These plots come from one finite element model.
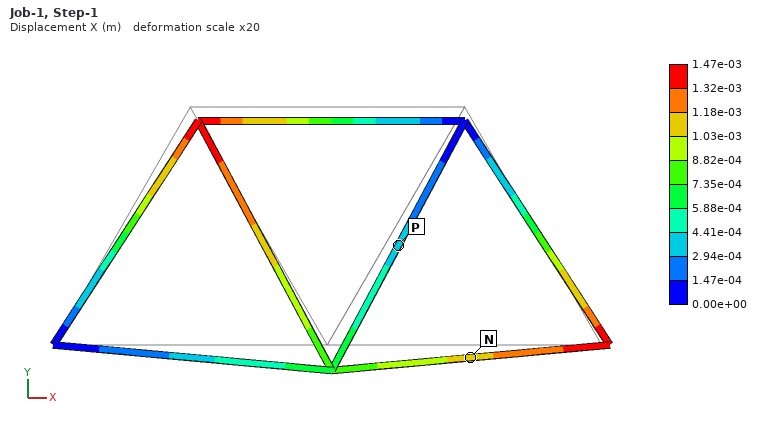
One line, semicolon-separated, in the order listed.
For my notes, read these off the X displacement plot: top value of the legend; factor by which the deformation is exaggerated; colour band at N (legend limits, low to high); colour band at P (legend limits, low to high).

1.47e-03 m; 20; 1.03e-03 to 1.18e-03 m; 2.94e-04 to 4.41e-04 m
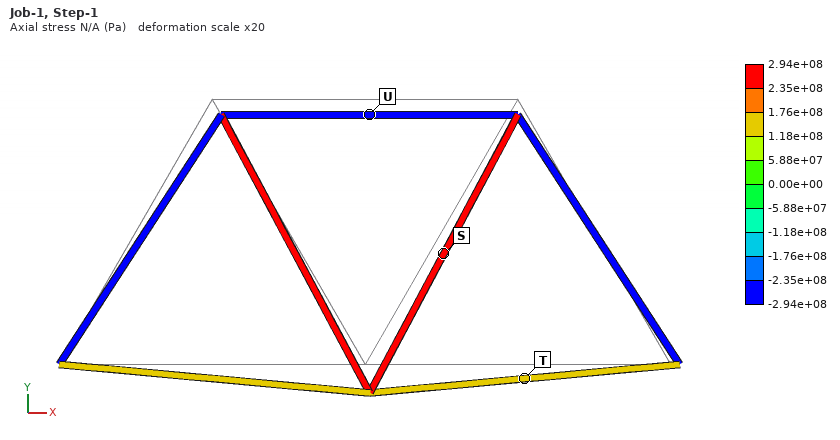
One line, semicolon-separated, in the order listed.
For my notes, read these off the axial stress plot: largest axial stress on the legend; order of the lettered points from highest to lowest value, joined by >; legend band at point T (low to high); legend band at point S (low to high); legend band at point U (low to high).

2.94e+08 Pa; S > T > U; 1.18e+08 to 1.76e+08 Pa; 2.35e+08 to 2.94e+08 Pa; -2.94e+08 to -2.35e+08 Pa
